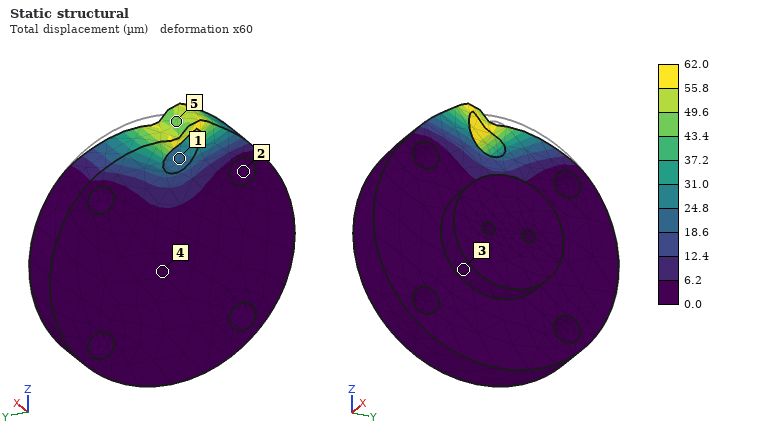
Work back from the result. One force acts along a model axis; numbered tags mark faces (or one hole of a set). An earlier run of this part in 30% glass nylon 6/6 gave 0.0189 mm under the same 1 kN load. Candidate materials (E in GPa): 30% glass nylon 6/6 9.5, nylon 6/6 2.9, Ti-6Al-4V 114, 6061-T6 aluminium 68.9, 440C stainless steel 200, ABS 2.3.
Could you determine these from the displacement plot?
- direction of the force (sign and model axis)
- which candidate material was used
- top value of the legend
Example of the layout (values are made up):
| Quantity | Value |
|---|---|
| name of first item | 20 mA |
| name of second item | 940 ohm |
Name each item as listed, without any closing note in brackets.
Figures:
| Quantity | Value |
|---|---|
| direction of the force | -Y |
| which candidate material was used | nylon 6/6 |
| top value of the legend | 62.0 µm |
